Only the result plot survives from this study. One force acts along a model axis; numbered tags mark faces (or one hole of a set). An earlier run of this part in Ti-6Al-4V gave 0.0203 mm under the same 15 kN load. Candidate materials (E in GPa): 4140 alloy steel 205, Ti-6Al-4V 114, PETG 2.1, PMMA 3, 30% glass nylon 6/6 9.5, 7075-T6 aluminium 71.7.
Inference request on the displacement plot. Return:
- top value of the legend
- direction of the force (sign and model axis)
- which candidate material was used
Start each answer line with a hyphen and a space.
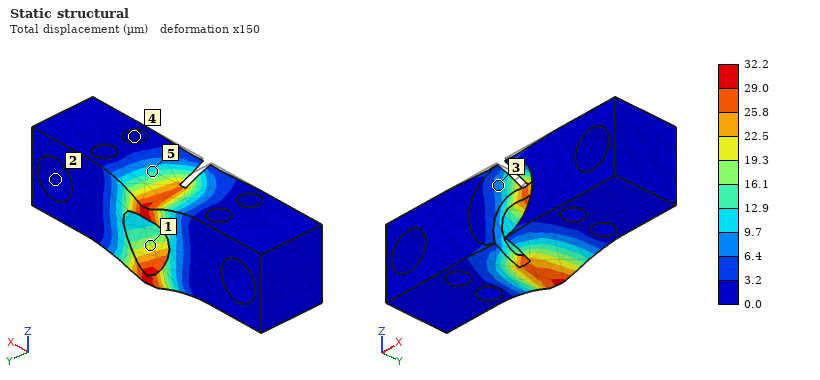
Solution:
- 32.2 µm
- -Z
- 7075-T6 aluminium
